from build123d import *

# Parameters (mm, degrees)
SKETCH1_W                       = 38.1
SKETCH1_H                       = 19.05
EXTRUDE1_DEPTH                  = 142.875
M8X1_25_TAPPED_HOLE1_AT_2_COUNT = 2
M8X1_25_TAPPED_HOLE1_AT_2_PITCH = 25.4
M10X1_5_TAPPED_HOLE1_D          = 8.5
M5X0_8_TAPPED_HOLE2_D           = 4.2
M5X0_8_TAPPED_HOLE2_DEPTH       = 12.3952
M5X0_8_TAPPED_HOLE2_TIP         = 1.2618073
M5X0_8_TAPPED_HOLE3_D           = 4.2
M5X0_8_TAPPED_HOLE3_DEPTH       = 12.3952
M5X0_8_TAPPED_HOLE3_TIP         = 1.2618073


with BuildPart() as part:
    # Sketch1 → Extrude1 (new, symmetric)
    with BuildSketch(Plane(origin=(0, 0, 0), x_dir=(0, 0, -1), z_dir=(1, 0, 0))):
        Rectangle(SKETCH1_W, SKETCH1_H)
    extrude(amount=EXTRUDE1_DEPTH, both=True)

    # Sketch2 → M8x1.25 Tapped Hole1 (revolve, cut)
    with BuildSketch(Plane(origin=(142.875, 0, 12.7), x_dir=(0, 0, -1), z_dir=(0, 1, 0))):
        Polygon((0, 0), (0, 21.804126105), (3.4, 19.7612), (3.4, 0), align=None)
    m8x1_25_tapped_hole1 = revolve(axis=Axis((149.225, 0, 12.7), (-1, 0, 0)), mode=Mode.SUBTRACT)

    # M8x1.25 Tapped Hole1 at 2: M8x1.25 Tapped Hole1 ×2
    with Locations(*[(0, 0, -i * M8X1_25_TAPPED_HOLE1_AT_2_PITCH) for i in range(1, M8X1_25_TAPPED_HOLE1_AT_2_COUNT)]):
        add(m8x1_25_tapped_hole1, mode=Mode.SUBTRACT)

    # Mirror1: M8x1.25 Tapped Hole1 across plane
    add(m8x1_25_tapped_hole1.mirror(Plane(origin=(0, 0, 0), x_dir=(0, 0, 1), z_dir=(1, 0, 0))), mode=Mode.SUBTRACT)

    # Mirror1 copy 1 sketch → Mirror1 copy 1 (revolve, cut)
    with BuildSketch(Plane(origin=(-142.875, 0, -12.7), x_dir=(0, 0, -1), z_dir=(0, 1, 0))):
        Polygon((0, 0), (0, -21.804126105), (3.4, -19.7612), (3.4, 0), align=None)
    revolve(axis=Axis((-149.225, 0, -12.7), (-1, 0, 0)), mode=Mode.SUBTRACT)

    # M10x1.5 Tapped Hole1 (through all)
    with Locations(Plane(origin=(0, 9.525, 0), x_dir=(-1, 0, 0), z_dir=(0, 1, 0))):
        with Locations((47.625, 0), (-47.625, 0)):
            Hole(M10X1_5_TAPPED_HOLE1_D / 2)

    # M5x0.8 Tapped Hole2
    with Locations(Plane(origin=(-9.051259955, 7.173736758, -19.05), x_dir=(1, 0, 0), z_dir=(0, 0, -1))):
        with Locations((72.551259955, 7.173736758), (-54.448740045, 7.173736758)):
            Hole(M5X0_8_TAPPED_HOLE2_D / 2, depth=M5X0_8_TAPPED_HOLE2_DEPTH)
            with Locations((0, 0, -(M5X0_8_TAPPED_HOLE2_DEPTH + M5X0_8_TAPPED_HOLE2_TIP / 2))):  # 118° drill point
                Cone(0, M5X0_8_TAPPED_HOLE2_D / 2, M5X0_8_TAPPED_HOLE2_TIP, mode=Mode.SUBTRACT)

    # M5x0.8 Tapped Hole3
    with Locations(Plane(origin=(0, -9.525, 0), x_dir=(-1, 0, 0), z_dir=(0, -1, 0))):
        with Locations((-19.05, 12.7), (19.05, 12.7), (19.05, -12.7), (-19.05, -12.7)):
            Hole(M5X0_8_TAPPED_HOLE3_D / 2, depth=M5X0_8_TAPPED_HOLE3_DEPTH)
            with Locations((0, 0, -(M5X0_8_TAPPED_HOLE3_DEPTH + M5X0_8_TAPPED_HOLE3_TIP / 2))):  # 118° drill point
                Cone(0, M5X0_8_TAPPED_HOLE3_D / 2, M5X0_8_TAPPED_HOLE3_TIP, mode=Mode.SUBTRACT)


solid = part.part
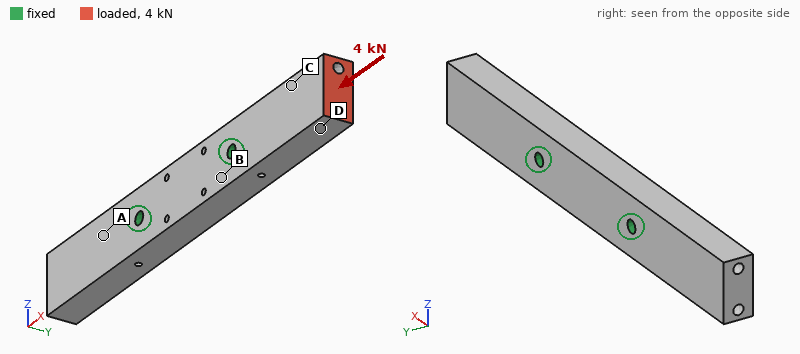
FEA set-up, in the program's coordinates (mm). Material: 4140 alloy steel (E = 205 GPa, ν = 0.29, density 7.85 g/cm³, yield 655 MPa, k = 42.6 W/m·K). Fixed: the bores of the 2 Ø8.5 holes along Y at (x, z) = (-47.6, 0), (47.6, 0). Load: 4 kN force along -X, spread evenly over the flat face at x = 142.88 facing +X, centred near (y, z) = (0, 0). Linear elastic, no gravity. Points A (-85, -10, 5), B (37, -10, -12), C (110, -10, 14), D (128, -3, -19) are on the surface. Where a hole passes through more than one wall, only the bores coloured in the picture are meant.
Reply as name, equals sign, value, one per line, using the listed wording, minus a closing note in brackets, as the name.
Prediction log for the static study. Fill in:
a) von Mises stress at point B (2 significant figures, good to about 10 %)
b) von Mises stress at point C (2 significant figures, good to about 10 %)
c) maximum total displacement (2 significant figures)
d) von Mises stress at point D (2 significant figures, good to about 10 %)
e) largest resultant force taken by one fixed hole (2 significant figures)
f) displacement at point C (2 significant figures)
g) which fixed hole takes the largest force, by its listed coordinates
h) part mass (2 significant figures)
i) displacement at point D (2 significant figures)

von Mises stress at point B = 1.9 MPa
von Mises stress at point C = 5.5 MPa
maximum total displacement = 2.9 µm
von Mises stress at point D = 6.4 MPa
largest resultant force taken by one fixed hole = 3.7 kN
displacement at point C = 1.8 µm
which fixed hole takes the largest force, by its listed coordinates = (47.6, 0)
part mass = 1.6 kg
displacement at point D = 2.4 µm
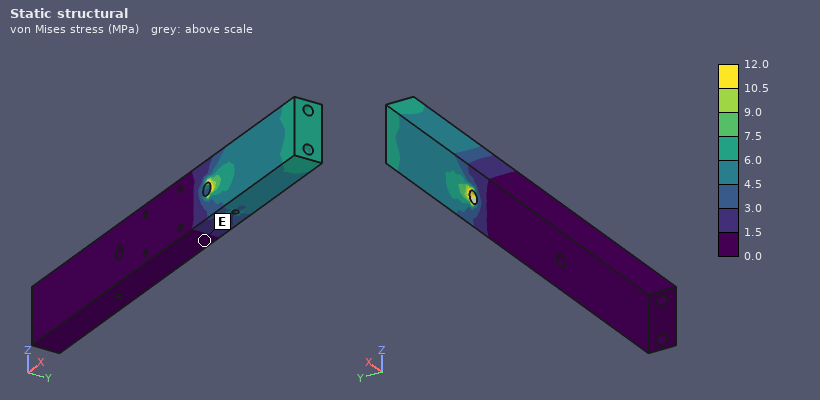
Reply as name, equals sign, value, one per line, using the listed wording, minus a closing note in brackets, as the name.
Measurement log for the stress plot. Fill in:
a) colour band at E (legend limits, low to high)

colour band at E = 0.0 to 1.5 MPa
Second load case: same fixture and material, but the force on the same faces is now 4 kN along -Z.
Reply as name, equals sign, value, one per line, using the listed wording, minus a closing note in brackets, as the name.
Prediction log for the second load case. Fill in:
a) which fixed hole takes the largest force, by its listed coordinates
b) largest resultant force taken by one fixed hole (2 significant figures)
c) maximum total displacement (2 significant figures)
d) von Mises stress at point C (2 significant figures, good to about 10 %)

which fixed hole takes the largest force, by its listed coordinates = (47.6, 0)
largest resultant force taken by one fixed hole = 6.6 kN
maximum total displacement = 0.12 mm
von Mises stress at point C = 22 MPa
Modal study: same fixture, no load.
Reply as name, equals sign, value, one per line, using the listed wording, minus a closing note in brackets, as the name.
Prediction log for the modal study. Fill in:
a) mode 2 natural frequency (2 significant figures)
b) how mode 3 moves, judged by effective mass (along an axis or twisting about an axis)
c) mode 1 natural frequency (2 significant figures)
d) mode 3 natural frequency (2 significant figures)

mode 2 natural frequency = 1700 Hz
how mode 3 moves, judged by effective mass = along Z
mode 1 natural frequency = 1700 Hz
mode 3 natural frequency = 2300 Hz
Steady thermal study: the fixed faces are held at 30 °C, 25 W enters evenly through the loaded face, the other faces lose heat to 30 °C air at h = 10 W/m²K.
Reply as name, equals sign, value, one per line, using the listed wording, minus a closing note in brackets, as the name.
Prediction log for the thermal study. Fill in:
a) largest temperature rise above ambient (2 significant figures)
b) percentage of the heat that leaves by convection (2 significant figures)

largest temperature rise above ambient = 71 K
percentage of the heat that leaves by convection = 18 %
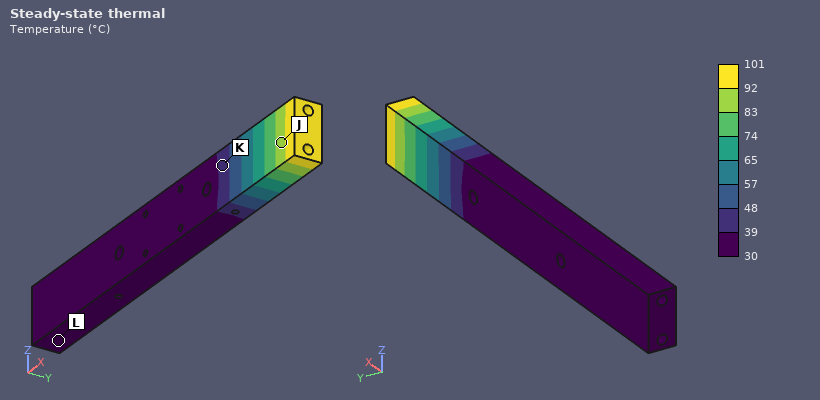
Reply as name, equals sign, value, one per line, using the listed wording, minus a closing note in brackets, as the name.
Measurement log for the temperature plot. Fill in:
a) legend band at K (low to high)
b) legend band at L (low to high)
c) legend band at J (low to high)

legend band at K = 39 to 48 °C
legend band at L = 30 to 39 °C
legend band at J = 83 to 92 °C
